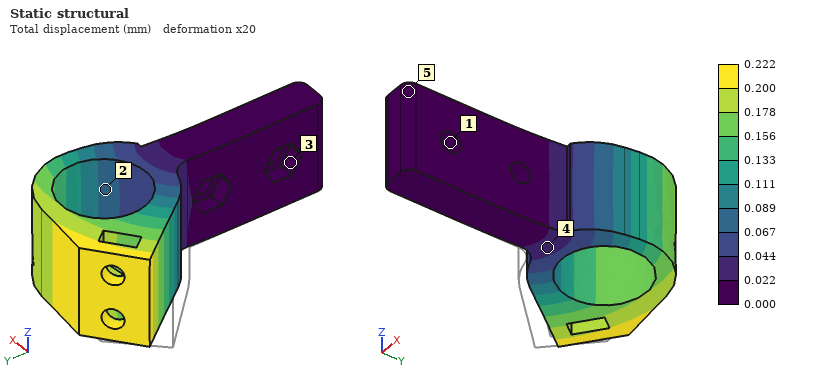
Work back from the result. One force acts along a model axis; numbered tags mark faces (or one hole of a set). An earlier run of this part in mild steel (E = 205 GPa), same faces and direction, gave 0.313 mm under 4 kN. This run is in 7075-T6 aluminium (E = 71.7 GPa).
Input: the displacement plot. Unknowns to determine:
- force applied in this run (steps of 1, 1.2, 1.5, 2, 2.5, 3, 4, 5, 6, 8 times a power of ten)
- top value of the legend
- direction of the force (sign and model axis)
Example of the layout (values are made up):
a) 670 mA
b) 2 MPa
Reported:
a) 1 kN
b) 0.222 mm
c) +X
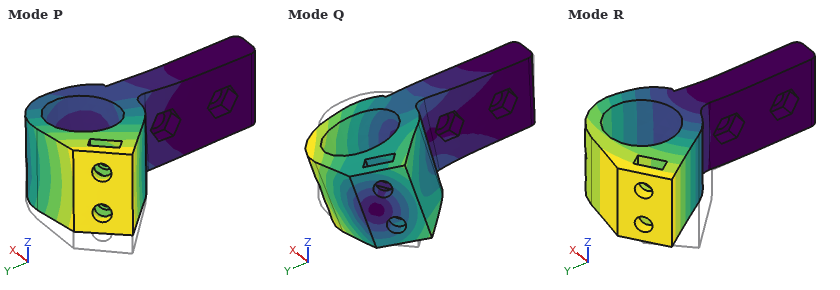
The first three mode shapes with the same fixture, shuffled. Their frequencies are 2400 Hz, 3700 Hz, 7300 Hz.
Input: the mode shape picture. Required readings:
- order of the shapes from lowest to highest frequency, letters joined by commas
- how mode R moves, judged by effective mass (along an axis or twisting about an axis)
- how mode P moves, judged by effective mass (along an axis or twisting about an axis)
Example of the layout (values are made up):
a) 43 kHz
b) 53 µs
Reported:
a) R, P, Q
b) along X
c) along Z
